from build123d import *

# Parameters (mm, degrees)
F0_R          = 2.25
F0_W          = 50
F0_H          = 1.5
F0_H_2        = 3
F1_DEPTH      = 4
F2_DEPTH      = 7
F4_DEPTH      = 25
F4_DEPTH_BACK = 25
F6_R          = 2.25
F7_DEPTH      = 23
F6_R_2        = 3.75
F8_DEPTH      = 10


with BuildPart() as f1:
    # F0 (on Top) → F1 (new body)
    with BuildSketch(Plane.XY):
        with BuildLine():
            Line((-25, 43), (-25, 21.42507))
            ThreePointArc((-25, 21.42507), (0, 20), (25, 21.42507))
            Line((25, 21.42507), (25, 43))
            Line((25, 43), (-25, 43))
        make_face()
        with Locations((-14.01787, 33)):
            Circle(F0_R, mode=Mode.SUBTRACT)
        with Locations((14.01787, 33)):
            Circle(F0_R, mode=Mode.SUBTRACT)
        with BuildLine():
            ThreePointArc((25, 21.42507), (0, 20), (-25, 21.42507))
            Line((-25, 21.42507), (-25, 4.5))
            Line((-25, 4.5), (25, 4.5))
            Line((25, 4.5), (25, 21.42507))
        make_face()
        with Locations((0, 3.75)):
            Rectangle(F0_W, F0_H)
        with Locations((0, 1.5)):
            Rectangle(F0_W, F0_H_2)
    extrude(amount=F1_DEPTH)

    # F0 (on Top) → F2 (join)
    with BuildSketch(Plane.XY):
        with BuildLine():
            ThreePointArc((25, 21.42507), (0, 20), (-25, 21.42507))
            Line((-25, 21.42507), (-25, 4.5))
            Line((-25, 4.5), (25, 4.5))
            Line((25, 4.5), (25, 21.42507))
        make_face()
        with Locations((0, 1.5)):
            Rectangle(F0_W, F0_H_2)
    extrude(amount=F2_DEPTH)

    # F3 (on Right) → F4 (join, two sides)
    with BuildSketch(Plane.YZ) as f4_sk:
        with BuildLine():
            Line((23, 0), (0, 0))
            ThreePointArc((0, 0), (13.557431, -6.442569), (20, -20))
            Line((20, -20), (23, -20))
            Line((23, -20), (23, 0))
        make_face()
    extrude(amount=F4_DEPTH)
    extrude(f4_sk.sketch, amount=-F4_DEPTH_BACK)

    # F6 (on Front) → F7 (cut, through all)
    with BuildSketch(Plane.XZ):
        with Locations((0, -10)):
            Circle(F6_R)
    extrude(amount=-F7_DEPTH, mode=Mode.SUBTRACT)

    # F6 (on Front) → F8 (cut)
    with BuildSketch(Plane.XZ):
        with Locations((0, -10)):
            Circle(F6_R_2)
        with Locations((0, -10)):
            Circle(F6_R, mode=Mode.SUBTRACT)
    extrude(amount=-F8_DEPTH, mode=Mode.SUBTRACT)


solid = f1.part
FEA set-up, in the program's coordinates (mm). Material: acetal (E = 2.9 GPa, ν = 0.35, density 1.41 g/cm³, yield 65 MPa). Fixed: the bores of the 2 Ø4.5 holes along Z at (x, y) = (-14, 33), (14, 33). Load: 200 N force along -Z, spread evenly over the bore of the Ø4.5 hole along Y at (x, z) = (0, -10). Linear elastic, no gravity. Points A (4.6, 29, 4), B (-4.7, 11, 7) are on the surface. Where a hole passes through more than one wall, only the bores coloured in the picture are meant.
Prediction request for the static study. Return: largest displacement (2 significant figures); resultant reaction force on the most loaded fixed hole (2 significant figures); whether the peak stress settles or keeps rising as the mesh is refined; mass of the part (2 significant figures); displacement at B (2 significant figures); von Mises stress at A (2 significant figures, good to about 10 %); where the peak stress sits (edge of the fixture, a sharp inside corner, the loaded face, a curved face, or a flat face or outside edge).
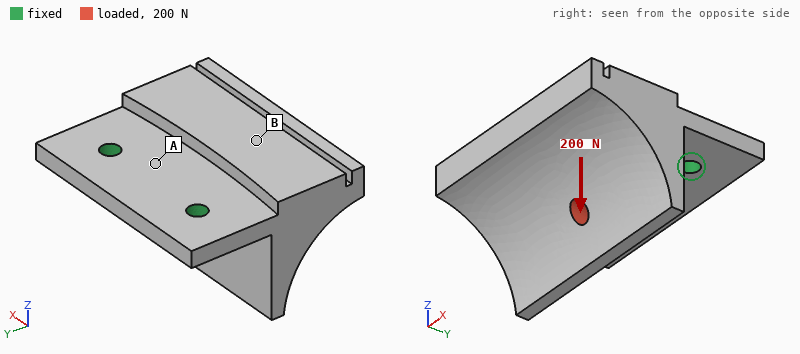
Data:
0.69 mm
100 N
keeps rising
27 g
0.44 mm
8.1 MPa
edge of the fixture
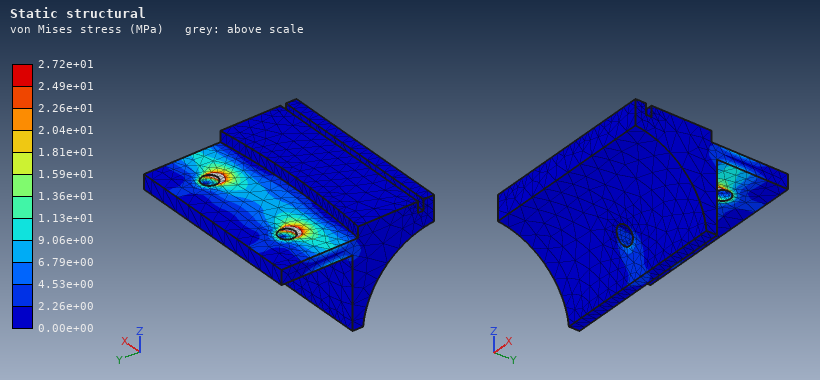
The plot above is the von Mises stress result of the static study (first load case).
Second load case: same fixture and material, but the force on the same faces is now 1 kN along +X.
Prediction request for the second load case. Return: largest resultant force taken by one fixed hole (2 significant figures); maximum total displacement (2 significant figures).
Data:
750 N
0.64 mm
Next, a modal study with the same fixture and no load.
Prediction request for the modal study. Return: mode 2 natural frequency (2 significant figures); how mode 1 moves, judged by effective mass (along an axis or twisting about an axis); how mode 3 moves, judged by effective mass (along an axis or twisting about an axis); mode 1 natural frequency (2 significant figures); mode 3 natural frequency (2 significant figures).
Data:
1600 Hz
along Z
along X
530 Hz
2800 Hz
